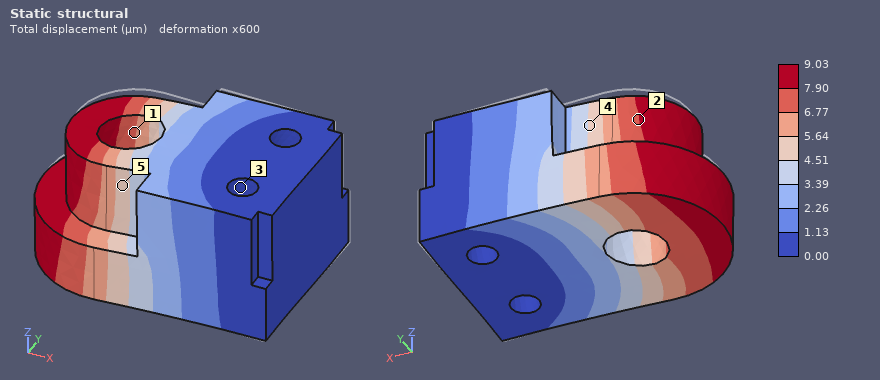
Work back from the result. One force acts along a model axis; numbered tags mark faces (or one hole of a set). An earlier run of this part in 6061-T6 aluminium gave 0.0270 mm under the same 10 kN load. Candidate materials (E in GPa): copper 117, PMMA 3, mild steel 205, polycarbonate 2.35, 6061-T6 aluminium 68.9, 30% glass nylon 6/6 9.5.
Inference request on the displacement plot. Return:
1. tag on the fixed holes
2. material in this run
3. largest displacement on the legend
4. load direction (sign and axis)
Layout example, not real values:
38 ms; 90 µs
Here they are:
3; mild steel; 9.03 µm; -Y
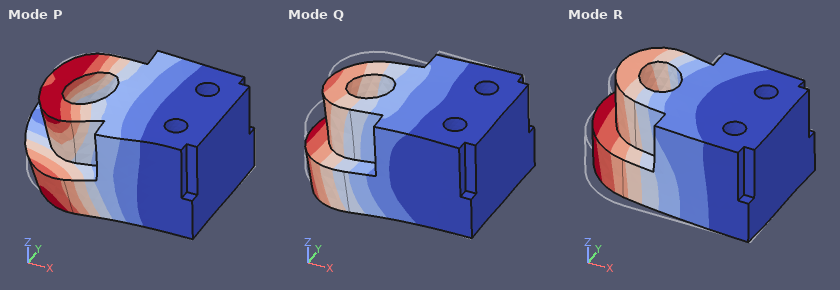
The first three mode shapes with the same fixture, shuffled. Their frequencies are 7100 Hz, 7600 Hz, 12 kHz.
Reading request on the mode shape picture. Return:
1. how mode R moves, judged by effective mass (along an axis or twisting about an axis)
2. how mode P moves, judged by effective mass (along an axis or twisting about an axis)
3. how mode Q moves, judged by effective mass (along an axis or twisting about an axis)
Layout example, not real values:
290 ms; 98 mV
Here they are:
along Y; twisting about X; along Z
